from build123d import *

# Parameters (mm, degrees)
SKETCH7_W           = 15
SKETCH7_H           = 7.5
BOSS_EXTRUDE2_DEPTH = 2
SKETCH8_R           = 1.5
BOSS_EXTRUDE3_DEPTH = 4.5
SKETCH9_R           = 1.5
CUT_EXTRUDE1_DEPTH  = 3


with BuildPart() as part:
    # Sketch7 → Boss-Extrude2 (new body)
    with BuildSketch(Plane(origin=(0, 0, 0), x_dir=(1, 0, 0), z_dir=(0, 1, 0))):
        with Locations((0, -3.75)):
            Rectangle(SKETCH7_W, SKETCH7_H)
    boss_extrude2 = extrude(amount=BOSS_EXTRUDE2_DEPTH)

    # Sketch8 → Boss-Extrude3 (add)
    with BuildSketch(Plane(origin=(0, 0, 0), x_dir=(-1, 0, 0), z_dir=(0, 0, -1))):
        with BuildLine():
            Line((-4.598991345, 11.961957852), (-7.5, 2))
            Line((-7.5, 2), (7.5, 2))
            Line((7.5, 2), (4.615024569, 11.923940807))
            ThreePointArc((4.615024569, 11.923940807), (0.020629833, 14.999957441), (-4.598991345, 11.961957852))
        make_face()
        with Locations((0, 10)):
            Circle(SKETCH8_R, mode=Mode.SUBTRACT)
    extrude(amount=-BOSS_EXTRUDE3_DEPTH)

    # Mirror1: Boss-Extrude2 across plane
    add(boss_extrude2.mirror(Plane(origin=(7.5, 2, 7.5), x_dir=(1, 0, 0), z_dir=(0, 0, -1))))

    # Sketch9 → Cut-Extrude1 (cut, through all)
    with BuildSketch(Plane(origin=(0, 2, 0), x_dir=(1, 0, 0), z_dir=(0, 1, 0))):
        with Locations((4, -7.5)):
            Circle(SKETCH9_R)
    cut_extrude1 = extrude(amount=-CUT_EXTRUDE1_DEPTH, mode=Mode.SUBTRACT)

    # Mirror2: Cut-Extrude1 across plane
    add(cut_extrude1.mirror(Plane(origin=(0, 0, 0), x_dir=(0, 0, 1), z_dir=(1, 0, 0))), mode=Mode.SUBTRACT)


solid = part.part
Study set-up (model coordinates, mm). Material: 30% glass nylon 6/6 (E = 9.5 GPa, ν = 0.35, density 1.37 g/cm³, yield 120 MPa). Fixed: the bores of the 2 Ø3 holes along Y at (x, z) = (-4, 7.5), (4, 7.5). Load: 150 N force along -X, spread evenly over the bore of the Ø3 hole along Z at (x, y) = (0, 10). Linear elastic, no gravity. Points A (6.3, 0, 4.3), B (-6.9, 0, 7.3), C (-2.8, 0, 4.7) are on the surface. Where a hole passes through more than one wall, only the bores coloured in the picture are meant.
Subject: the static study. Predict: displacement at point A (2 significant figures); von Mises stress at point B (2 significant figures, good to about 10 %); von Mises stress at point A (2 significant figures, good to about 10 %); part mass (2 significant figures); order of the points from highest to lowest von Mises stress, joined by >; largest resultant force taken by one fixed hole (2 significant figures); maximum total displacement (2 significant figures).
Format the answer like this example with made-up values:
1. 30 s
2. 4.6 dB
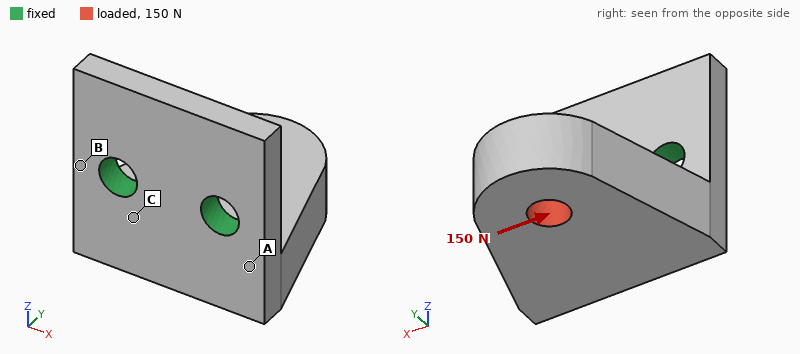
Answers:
1. 25 µm
2. 25 MPa
3. 14 MPa
4. 1.4 g
5. B > A > C
6. 170 N
7. 93 µm
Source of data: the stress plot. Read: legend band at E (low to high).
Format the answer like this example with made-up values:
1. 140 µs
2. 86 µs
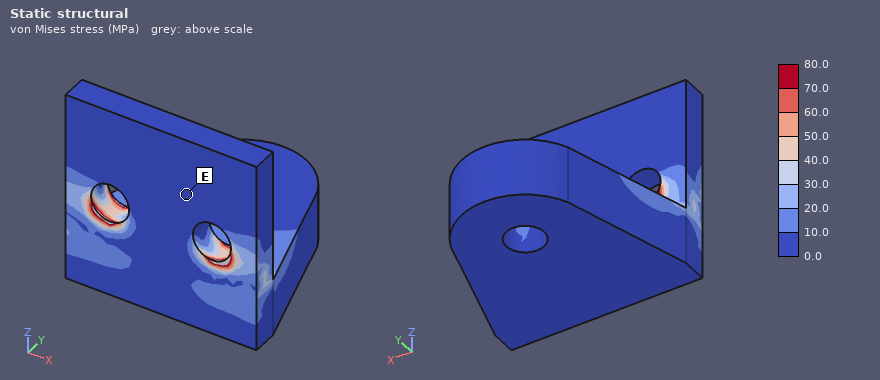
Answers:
1. 0.0 to 10.0 MPa
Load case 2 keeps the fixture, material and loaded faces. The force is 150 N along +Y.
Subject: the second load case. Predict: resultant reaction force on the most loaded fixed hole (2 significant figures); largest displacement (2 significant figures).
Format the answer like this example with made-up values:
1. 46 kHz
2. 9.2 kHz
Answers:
1. 75 N
2. 0.21 mm
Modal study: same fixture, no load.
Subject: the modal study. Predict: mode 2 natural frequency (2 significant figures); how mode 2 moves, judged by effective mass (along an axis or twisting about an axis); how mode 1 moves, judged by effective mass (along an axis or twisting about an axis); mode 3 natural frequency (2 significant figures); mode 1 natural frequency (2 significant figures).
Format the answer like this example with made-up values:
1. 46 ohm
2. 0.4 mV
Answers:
1. 9700 Hz
2. along X
3. along Z
4. 18 kHz
5. 3800 Hz
